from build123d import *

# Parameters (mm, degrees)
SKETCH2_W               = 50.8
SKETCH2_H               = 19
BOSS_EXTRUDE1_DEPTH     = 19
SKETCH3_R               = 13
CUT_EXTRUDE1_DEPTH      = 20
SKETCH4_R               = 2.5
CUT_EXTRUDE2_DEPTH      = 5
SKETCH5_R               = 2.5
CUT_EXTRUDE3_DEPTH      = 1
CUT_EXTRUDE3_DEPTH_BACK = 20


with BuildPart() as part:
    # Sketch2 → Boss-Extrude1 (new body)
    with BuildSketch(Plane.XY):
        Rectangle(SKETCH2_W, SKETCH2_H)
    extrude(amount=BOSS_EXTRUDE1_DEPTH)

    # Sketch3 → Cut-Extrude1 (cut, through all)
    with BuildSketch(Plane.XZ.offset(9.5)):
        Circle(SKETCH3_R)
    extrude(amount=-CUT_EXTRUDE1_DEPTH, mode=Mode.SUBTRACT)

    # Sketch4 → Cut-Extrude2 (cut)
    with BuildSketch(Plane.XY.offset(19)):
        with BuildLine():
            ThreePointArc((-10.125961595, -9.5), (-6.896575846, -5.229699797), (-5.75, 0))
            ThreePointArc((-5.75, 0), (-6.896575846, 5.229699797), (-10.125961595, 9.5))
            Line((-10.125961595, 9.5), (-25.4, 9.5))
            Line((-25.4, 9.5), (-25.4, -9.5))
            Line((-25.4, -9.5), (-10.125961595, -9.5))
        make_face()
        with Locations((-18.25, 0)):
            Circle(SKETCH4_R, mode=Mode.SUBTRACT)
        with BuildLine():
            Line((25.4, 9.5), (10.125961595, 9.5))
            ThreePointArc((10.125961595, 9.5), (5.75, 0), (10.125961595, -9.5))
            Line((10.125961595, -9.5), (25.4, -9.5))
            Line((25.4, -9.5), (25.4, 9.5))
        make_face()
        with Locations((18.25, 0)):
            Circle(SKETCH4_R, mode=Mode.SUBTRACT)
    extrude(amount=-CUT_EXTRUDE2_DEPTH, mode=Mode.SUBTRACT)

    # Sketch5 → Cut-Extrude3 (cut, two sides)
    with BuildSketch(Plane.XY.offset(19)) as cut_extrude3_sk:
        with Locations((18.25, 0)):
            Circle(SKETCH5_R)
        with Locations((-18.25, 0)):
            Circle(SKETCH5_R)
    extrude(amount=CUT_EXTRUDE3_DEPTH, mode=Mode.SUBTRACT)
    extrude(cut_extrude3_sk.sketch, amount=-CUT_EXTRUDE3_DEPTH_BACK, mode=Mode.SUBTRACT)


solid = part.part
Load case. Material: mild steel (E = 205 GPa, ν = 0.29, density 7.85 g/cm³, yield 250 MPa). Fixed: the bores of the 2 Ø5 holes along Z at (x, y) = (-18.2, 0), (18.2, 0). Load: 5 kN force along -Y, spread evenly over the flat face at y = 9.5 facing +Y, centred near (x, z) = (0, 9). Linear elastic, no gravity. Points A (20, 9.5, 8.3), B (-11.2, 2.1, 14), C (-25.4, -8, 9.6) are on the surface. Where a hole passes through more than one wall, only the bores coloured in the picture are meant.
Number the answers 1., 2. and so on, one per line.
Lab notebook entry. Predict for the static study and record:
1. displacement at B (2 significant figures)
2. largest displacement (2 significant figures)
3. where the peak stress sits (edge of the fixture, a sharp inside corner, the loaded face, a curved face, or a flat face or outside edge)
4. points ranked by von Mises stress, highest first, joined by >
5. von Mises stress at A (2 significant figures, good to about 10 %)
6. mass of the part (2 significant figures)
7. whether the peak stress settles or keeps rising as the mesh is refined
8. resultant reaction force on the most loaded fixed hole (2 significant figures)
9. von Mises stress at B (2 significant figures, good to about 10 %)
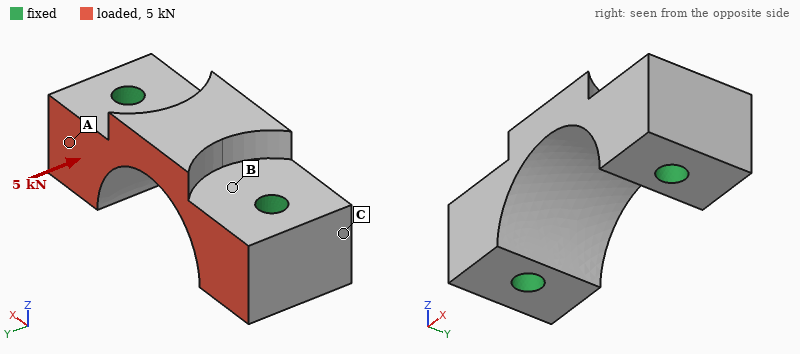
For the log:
1. 1.5 µm
2. 6.9 µm
3. edge of the fixture
4. B > A > C
5. 15 MPa
6. 73 g
7. keeps rising
8. 2.5 kN
9. 26 MPa
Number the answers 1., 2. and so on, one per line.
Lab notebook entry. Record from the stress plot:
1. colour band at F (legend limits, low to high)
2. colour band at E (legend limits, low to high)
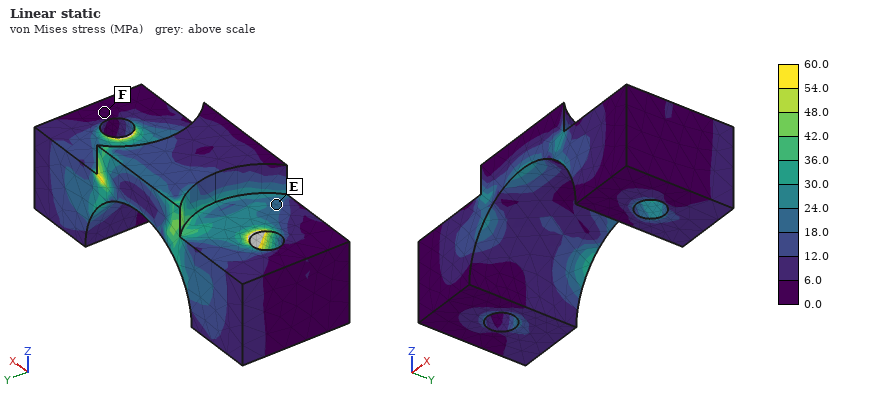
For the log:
1. 0.0 to 6.0 MPa
2. 18.0 to 24.0 MPa
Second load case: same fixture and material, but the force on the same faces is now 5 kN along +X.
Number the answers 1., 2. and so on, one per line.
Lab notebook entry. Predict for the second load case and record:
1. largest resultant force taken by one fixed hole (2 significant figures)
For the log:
1. 2.6 kN
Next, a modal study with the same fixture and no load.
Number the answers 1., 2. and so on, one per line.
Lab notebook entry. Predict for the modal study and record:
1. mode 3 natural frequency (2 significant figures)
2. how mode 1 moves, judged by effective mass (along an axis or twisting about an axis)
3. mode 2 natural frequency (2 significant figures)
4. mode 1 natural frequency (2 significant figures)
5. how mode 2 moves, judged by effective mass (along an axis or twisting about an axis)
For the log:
1. 45 kHz
2. along Y
3. 34 kHz
4. 23 kHz
5. along Z
